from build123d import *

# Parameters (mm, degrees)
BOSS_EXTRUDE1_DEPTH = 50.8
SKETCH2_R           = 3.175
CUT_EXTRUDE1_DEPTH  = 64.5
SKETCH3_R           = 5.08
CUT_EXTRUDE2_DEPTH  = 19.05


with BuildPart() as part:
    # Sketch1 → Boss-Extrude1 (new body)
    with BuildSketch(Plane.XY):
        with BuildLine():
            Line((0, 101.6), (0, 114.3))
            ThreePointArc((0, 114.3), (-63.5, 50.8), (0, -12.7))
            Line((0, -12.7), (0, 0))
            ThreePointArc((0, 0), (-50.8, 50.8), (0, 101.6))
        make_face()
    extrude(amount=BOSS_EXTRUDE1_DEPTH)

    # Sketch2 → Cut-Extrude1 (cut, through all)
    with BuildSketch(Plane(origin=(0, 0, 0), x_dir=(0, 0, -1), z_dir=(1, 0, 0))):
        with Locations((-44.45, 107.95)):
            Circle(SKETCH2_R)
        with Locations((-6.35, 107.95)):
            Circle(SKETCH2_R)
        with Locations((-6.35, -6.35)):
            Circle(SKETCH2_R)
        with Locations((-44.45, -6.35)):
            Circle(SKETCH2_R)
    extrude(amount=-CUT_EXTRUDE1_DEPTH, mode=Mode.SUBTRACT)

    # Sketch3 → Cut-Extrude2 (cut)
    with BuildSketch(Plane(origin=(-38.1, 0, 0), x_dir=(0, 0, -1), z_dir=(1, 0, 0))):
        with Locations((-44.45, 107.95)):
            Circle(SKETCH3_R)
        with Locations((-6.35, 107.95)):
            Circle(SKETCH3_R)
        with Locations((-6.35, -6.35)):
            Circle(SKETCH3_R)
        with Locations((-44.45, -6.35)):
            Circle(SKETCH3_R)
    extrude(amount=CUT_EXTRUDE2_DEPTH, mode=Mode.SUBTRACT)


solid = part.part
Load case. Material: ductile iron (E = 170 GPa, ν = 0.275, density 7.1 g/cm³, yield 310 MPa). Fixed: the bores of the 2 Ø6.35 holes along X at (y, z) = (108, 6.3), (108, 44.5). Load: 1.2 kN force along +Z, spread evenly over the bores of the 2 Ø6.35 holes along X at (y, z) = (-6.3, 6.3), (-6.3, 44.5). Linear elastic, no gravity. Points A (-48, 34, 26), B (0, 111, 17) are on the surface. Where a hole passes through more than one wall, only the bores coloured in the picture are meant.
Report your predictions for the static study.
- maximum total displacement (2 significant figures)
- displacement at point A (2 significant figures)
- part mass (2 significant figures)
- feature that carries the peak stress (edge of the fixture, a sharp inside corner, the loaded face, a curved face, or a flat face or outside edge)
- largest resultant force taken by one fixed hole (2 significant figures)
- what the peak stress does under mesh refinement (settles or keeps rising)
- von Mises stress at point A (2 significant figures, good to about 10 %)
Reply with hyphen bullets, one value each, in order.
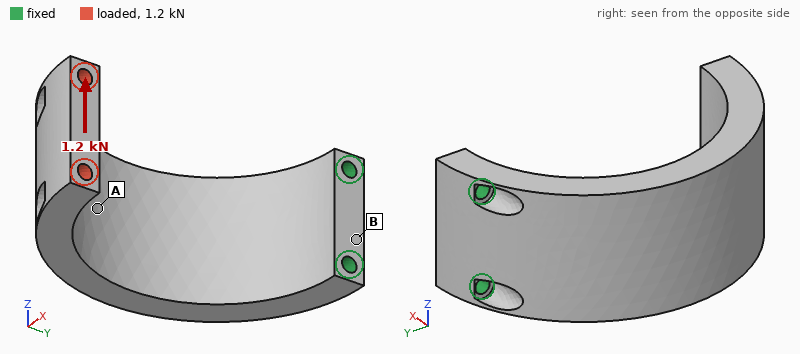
- 0.40 mm
- 0.13 mm
- 790 g
- edge of the fixture
- 3.5 kN
- keeps rising
- 33 MPa
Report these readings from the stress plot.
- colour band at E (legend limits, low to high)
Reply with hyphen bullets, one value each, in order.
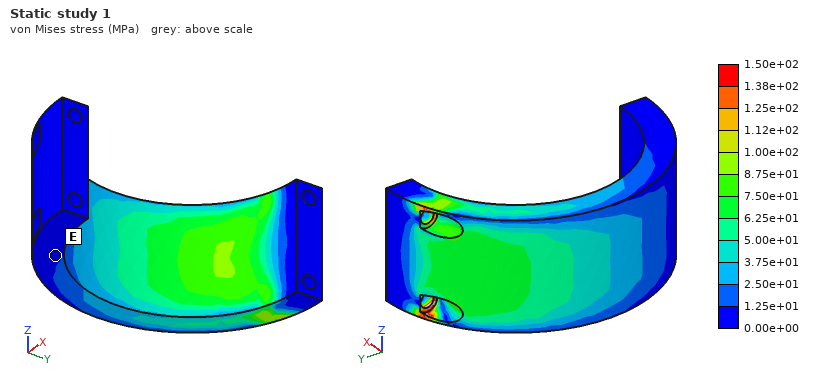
- 0.00e+00 to 1.25e+01 MPa
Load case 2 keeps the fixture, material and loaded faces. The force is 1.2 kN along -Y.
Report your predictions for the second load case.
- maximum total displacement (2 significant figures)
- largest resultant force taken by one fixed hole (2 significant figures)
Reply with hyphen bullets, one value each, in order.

- 0.32 mm
- 610 N
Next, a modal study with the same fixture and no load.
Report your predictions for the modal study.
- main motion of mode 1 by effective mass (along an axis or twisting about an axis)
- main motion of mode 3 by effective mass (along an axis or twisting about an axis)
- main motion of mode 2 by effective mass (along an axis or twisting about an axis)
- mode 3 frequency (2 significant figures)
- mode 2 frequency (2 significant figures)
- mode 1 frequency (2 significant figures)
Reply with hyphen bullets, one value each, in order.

- along X
- along Y
- along Z
- 1300 Hz
- 680 Hz
- 400 Hz
